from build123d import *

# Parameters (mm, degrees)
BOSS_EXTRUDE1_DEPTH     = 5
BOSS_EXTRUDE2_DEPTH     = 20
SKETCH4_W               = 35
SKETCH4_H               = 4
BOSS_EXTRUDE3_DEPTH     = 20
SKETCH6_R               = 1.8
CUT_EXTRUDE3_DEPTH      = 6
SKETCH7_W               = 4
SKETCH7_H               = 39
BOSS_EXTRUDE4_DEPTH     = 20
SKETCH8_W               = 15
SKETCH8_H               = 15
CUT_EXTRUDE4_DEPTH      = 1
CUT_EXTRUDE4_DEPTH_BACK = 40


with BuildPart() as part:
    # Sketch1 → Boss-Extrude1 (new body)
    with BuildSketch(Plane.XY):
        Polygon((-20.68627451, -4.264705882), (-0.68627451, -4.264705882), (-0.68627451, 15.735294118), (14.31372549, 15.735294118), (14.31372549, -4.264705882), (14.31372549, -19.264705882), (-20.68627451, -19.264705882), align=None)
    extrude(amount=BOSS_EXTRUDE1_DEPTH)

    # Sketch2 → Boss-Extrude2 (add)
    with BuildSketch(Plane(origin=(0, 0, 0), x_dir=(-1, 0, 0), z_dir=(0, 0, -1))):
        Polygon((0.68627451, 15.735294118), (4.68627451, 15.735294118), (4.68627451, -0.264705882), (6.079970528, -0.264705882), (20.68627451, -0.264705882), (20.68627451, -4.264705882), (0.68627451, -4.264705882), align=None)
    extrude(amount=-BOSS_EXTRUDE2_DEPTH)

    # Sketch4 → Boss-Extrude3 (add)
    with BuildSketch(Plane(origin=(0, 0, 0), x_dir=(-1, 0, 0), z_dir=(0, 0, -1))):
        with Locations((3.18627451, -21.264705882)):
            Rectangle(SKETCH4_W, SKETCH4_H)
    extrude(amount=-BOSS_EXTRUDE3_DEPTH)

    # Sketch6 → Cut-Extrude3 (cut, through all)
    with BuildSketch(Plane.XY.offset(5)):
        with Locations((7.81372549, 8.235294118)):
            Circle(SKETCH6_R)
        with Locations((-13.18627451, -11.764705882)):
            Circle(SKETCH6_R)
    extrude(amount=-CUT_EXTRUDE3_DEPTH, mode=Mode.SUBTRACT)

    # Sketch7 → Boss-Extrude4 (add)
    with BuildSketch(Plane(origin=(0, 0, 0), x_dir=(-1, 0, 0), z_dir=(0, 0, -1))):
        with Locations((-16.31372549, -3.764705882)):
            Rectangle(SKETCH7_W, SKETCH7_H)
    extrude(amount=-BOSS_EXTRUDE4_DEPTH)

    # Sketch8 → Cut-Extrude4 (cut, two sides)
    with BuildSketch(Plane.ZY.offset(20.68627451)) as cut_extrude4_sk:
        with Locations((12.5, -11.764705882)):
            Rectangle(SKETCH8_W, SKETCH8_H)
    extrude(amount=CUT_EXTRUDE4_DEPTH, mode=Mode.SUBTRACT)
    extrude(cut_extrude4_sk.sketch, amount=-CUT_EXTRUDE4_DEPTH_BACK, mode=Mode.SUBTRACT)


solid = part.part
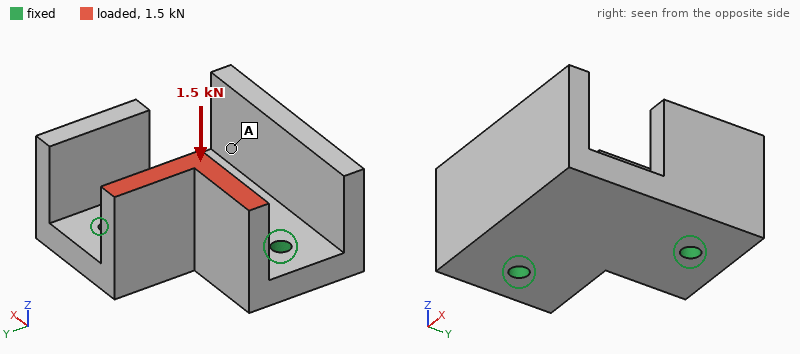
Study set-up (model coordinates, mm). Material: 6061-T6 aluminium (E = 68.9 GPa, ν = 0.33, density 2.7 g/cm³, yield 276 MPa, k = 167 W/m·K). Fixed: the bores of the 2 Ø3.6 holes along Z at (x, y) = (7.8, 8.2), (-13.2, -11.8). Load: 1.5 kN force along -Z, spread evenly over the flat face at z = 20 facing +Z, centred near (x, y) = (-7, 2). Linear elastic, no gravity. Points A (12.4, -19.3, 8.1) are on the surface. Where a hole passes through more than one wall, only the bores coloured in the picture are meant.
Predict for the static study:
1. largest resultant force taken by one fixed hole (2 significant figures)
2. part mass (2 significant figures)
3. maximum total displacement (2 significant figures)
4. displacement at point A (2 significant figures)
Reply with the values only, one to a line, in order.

790 N
32 g
41 µm
9.0 µm
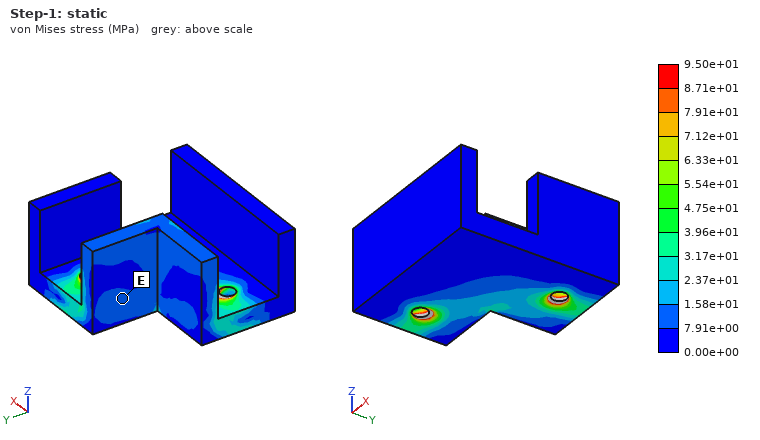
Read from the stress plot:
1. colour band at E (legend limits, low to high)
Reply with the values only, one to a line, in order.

7.91e+00 to 1.58e+01 MPa
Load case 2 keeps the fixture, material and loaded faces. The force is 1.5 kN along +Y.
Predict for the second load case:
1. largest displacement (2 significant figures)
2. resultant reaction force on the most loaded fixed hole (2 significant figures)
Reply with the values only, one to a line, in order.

0.17 mm
1.1 kN
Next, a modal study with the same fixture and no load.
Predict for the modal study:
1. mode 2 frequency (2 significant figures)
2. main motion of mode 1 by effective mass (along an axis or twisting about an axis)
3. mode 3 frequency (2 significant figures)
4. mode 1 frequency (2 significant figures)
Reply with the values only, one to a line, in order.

7500 Hz
along Z
8400 Hz
4500 Hz
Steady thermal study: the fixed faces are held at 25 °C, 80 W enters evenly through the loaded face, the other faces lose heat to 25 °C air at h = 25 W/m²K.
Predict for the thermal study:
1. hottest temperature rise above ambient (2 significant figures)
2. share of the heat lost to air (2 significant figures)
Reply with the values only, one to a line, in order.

78 K
3.5 %
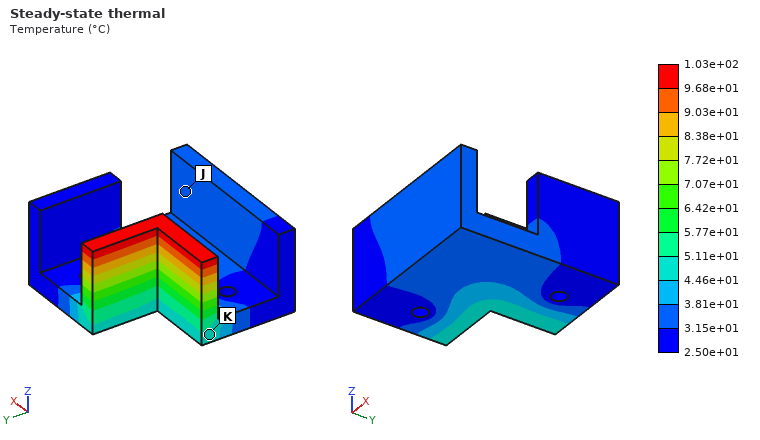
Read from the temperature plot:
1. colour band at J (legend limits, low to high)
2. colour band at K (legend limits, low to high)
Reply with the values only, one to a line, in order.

3.15e+01 to 3.81e+01 °C
4.46e+01 to 5.11e+01 °C
